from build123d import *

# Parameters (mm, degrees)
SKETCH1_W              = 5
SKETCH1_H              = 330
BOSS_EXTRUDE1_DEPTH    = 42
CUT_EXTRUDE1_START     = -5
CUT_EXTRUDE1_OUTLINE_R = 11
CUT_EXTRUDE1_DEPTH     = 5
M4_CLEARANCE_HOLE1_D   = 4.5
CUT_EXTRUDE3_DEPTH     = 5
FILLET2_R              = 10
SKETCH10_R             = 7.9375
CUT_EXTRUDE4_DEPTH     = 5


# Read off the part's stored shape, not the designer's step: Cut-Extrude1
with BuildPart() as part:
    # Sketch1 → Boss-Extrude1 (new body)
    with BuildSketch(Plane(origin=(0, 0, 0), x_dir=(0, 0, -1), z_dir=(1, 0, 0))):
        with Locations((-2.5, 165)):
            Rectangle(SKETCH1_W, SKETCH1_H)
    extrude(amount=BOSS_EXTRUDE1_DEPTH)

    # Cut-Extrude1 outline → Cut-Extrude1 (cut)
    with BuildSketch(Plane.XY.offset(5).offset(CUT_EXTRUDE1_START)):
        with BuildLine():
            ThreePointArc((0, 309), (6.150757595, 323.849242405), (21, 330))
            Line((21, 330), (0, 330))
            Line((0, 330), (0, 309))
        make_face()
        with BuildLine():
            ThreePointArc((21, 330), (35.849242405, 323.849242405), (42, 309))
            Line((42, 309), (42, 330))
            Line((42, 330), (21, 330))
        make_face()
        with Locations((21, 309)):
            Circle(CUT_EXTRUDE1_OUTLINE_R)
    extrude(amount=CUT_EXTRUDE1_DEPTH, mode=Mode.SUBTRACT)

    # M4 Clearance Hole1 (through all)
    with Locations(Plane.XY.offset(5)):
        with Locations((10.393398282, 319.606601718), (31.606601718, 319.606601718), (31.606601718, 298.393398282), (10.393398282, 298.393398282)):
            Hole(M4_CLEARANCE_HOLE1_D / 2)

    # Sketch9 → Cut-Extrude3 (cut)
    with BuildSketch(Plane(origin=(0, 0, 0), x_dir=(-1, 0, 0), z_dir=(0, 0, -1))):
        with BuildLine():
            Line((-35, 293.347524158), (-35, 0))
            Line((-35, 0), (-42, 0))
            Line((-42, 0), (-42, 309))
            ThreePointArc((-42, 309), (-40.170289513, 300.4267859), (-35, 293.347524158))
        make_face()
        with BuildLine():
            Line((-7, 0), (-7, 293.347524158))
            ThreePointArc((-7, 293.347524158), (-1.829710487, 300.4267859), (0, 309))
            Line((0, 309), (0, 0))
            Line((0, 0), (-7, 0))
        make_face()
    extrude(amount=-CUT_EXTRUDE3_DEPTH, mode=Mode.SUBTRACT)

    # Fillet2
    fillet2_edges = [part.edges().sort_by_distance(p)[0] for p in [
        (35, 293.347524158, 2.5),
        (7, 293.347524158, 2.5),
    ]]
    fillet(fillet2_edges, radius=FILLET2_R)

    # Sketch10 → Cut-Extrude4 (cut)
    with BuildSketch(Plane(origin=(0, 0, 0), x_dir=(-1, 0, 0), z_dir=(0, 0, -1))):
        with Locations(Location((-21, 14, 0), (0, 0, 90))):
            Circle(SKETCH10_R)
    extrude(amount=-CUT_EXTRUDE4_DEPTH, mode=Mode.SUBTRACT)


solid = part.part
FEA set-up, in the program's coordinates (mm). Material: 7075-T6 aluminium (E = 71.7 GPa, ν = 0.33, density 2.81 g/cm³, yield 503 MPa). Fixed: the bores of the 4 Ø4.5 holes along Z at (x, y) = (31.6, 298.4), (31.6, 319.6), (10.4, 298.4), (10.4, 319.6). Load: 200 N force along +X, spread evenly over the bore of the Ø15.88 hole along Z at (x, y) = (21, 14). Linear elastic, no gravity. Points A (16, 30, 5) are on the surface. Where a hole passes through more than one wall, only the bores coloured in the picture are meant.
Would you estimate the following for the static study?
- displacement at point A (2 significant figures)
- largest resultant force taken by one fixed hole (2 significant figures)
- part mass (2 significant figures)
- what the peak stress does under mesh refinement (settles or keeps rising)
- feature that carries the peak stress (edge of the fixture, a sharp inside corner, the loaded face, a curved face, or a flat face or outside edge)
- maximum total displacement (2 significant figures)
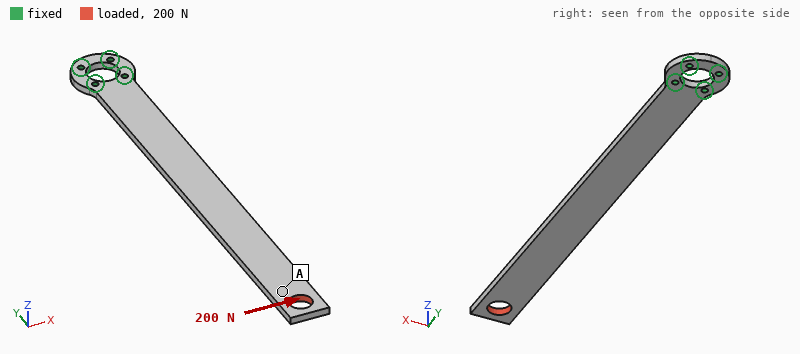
2.1 mm
2.4 kN
120 g
keeps rising
edge of the fixture
2.5 mm
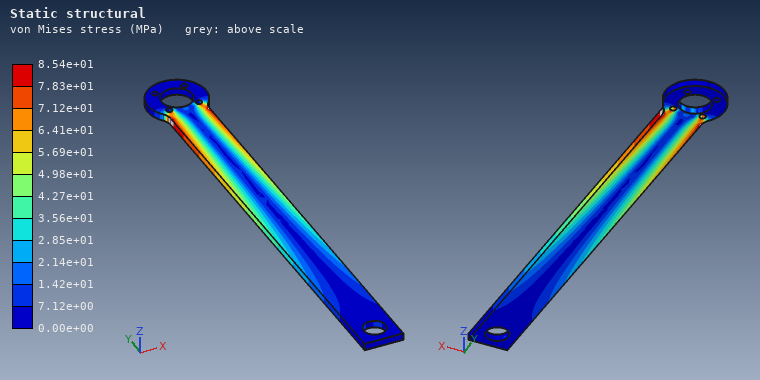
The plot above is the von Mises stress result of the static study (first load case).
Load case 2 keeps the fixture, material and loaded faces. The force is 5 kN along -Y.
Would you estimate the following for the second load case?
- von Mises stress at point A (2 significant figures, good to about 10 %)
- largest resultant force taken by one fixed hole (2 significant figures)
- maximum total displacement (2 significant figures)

32 MPa
2.6 kN
0.16 mm
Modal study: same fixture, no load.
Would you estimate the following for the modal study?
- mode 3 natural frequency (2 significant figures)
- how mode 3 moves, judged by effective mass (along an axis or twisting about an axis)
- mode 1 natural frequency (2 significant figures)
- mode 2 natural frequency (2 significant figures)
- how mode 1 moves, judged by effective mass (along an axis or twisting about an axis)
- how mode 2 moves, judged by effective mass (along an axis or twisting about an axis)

300 Hz
along Z
48 Hz
270 Hz
along Z
along X
